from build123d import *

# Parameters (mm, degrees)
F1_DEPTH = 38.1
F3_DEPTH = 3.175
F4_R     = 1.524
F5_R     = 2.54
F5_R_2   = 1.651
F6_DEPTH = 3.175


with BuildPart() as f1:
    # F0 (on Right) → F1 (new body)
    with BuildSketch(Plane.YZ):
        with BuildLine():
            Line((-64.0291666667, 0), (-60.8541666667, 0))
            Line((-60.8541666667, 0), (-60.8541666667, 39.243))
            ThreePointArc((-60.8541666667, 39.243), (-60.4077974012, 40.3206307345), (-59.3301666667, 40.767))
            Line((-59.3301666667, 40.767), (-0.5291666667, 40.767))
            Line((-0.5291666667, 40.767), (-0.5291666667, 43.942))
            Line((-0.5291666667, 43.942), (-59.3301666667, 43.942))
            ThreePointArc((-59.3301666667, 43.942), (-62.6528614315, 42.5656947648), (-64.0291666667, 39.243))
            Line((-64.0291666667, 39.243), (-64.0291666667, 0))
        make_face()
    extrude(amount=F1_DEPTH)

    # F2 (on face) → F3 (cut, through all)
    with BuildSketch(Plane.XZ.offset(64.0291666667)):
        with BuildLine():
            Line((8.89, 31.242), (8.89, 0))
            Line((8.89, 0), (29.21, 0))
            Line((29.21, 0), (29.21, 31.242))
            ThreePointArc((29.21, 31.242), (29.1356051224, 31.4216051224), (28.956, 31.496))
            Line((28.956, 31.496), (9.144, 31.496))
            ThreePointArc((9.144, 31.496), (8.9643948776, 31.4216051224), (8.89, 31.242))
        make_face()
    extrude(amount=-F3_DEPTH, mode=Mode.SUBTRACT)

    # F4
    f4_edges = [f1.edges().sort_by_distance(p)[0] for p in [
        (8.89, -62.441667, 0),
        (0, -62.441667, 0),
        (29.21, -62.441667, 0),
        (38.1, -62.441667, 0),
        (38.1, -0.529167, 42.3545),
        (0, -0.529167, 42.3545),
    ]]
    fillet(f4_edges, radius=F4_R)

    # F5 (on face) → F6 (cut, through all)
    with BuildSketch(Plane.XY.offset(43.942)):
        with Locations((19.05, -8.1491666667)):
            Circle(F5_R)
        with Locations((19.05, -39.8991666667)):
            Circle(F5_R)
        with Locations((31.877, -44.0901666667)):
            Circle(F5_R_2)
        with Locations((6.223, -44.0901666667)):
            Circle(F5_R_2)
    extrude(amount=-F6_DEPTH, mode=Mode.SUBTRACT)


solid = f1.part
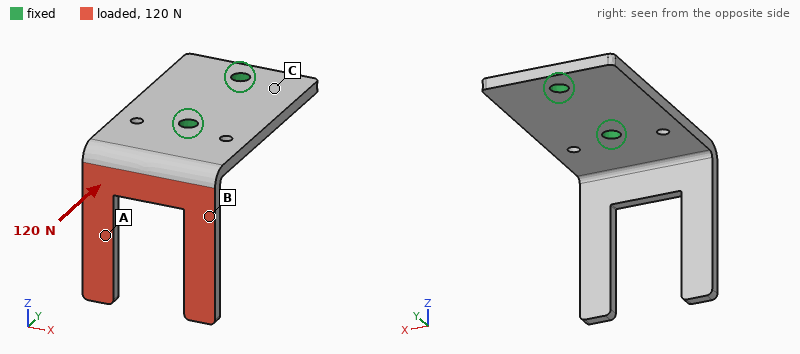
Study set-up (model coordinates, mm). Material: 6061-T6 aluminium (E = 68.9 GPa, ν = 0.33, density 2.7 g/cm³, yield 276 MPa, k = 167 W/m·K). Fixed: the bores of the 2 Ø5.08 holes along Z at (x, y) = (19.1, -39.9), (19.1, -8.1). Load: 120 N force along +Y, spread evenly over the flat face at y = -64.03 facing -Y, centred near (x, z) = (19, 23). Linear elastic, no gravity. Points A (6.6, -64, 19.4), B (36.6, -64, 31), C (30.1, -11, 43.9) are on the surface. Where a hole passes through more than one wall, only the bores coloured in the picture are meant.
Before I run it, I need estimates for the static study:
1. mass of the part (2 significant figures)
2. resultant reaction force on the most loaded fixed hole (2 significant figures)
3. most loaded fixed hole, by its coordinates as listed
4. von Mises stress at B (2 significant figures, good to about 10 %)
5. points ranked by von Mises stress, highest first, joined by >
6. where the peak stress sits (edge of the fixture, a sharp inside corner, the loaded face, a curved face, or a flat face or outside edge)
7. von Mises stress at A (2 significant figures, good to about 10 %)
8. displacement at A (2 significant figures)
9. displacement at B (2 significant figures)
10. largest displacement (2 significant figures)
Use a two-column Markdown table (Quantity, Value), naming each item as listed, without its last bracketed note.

| Quantity | Value |
|---|---|
| mass of the part | 28 g |
| resultant reaction force on the most loaded fixed hole | 100 N |
| most loaded fixed hole, by its coordinates as listed | (19.1, -39.9) |
| von Mises stress at B | 35 MPa |
| points ranked by von Mises stress, highest first, joined by > | B > A > C |
| where the peak stress sits | the loaded face |
| von Mises stress at A | 16 MPa |
| displacement at A | 0.27 mm |
| displacement at B | 0.15 mm |
| largest displacement | 0.55 mm |
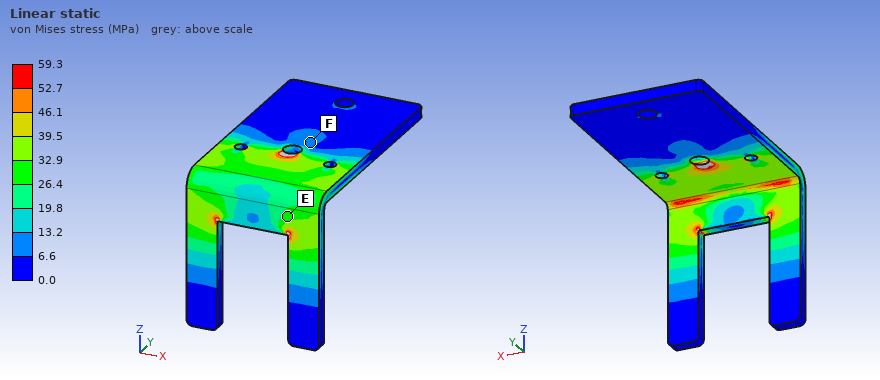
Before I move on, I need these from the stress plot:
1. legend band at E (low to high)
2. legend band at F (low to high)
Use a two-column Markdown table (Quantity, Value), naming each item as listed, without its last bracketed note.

| Quantity | Value |
|---|---|
| legend band at E | 26.4 to 32.9 MPa |
| legend band at F | 6.6 to 13.2 MPa |
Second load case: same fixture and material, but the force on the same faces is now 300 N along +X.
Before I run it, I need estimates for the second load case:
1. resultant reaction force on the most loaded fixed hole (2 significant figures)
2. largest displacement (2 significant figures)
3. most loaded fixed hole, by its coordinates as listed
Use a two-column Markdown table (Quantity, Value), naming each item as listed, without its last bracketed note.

| Quantity | Value |
|---|---|
| resultant reaction force on the most loaded fixed hole | 480 N |
| largest displacement | 0.60 mm |
| most loaded fixed hole, by its coordinates as listed | (19.1, -39.9) |
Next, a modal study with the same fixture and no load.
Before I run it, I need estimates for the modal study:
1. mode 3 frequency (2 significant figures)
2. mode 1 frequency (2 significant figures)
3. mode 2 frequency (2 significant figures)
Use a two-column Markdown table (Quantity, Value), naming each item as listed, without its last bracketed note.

| Quantity | Value |
|---|---|
| mode 3 frequency | 1700 Hz |
| mode 1 frequency | 1000 Hz |
| mode 2 frequency | 1300 Hz |
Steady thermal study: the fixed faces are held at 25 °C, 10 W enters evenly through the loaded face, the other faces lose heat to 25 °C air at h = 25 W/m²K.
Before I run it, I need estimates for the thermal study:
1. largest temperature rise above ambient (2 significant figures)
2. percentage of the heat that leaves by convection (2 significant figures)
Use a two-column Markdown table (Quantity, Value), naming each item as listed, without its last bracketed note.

| Quantity | Value |
|---|---|
| largest temperature rise above ambient | 27 K |
| percentage of the heat that leaves by convection | 12 % |
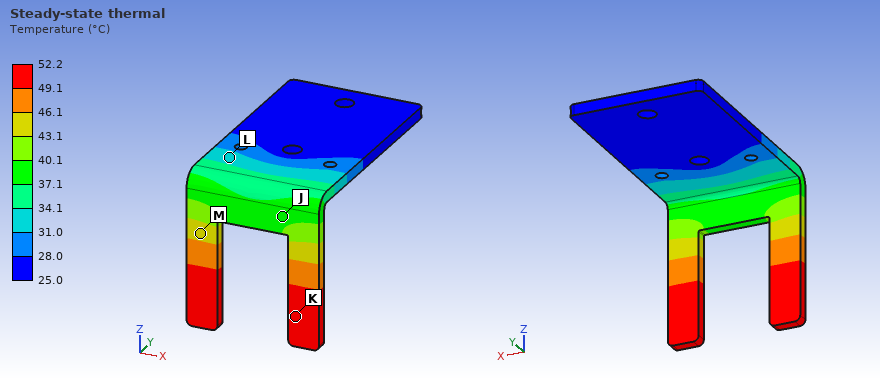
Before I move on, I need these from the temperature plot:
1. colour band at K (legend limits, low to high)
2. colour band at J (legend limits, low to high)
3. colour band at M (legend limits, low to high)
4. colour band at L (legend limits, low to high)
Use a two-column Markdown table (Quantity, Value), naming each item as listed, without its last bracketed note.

| Quantity | Value |
|---|---|
| colour band at K | 49.1 to 52.2 °C |
| colour band at J | 37.1 to 40.1 °C |
| colour band at M | 43.1 to 46.1 °C |
| colour band at L | 31.0 to 34.1 °C |
